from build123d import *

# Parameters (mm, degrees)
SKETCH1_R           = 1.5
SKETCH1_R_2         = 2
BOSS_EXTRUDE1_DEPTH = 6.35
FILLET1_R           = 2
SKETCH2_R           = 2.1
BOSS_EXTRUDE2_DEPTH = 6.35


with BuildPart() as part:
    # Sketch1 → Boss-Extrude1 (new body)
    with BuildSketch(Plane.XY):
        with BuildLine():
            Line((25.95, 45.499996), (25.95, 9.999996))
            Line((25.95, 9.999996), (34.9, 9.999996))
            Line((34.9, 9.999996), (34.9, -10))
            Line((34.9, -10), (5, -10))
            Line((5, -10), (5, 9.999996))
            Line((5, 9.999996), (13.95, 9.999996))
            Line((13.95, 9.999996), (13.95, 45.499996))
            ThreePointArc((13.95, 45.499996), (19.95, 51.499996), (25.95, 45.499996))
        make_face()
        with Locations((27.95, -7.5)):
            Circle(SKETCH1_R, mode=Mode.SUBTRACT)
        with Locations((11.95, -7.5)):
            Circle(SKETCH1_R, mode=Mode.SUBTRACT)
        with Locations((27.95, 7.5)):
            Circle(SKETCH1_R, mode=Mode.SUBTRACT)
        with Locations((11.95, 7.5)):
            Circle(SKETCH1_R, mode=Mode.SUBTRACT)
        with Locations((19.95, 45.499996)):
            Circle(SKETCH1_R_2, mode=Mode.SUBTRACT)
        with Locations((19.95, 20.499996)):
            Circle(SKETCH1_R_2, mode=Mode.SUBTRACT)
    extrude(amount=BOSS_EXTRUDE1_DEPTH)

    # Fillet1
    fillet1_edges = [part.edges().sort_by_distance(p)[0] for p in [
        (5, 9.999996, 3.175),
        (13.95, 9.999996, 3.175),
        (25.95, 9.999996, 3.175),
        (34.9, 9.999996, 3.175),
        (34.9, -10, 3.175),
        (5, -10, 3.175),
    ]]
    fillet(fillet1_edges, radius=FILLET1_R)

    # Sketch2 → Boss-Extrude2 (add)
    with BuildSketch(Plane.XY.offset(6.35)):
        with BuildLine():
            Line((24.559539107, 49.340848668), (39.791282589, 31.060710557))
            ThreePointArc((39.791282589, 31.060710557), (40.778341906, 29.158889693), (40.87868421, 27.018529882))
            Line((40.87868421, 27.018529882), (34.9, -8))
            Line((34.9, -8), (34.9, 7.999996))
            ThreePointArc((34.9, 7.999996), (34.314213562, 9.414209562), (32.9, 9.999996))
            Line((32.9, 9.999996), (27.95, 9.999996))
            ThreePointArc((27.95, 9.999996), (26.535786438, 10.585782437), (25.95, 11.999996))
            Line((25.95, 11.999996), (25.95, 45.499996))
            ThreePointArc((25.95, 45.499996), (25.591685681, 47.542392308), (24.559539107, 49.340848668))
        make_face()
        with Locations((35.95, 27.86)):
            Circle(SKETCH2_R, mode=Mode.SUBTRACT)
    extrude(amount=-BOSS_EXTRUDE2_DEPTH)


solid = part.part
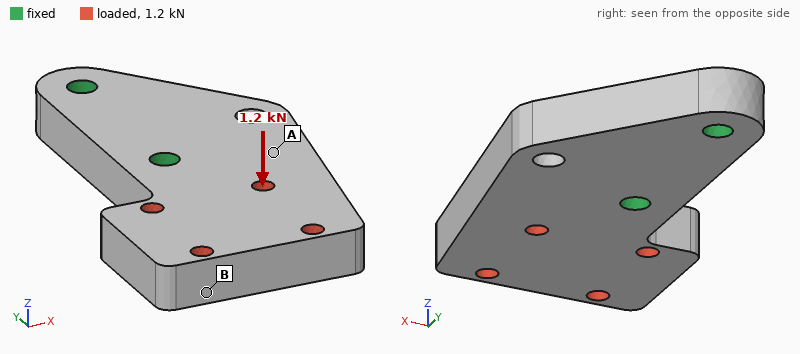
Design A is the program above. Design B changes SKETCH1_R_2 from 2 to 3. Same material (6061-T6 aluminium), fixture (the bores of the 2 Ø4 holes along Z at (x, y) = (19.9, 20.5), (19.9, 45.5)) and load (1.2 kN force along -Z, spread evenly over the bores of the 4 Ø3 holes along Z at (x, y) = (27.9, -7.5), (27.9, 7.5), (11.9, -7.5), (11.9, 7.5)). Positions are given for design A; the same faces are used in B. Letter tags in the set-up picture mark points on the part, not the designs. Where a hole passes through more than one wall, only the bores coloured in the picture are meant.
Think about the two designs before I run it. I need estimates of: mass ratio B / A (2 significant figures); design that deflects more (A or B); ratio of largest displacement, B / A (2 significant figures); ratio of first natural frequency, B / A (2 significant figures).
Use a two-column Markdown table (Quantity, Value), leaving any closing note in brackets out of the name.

| Quantity | Value |
|---|---|
| mass ratio B / A | 0.98 |
| design that deflects more | A |
| ratio of largest displacement, B / A | 0.85 |
| ratio of first natural frequency, B / A | 1.1 |
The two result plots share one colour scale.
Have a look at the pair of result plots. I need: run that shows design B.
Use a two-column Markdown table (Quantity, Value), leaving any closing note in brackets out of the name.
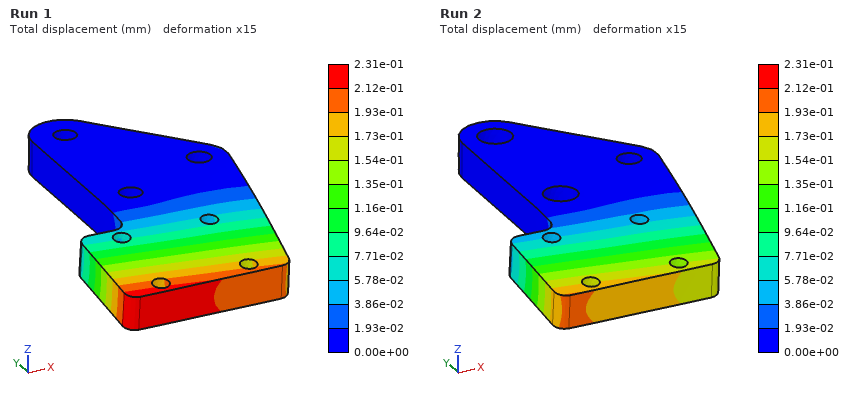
| Quantity | Value |
|---|---|
| run that shows design B | Run 2 |
